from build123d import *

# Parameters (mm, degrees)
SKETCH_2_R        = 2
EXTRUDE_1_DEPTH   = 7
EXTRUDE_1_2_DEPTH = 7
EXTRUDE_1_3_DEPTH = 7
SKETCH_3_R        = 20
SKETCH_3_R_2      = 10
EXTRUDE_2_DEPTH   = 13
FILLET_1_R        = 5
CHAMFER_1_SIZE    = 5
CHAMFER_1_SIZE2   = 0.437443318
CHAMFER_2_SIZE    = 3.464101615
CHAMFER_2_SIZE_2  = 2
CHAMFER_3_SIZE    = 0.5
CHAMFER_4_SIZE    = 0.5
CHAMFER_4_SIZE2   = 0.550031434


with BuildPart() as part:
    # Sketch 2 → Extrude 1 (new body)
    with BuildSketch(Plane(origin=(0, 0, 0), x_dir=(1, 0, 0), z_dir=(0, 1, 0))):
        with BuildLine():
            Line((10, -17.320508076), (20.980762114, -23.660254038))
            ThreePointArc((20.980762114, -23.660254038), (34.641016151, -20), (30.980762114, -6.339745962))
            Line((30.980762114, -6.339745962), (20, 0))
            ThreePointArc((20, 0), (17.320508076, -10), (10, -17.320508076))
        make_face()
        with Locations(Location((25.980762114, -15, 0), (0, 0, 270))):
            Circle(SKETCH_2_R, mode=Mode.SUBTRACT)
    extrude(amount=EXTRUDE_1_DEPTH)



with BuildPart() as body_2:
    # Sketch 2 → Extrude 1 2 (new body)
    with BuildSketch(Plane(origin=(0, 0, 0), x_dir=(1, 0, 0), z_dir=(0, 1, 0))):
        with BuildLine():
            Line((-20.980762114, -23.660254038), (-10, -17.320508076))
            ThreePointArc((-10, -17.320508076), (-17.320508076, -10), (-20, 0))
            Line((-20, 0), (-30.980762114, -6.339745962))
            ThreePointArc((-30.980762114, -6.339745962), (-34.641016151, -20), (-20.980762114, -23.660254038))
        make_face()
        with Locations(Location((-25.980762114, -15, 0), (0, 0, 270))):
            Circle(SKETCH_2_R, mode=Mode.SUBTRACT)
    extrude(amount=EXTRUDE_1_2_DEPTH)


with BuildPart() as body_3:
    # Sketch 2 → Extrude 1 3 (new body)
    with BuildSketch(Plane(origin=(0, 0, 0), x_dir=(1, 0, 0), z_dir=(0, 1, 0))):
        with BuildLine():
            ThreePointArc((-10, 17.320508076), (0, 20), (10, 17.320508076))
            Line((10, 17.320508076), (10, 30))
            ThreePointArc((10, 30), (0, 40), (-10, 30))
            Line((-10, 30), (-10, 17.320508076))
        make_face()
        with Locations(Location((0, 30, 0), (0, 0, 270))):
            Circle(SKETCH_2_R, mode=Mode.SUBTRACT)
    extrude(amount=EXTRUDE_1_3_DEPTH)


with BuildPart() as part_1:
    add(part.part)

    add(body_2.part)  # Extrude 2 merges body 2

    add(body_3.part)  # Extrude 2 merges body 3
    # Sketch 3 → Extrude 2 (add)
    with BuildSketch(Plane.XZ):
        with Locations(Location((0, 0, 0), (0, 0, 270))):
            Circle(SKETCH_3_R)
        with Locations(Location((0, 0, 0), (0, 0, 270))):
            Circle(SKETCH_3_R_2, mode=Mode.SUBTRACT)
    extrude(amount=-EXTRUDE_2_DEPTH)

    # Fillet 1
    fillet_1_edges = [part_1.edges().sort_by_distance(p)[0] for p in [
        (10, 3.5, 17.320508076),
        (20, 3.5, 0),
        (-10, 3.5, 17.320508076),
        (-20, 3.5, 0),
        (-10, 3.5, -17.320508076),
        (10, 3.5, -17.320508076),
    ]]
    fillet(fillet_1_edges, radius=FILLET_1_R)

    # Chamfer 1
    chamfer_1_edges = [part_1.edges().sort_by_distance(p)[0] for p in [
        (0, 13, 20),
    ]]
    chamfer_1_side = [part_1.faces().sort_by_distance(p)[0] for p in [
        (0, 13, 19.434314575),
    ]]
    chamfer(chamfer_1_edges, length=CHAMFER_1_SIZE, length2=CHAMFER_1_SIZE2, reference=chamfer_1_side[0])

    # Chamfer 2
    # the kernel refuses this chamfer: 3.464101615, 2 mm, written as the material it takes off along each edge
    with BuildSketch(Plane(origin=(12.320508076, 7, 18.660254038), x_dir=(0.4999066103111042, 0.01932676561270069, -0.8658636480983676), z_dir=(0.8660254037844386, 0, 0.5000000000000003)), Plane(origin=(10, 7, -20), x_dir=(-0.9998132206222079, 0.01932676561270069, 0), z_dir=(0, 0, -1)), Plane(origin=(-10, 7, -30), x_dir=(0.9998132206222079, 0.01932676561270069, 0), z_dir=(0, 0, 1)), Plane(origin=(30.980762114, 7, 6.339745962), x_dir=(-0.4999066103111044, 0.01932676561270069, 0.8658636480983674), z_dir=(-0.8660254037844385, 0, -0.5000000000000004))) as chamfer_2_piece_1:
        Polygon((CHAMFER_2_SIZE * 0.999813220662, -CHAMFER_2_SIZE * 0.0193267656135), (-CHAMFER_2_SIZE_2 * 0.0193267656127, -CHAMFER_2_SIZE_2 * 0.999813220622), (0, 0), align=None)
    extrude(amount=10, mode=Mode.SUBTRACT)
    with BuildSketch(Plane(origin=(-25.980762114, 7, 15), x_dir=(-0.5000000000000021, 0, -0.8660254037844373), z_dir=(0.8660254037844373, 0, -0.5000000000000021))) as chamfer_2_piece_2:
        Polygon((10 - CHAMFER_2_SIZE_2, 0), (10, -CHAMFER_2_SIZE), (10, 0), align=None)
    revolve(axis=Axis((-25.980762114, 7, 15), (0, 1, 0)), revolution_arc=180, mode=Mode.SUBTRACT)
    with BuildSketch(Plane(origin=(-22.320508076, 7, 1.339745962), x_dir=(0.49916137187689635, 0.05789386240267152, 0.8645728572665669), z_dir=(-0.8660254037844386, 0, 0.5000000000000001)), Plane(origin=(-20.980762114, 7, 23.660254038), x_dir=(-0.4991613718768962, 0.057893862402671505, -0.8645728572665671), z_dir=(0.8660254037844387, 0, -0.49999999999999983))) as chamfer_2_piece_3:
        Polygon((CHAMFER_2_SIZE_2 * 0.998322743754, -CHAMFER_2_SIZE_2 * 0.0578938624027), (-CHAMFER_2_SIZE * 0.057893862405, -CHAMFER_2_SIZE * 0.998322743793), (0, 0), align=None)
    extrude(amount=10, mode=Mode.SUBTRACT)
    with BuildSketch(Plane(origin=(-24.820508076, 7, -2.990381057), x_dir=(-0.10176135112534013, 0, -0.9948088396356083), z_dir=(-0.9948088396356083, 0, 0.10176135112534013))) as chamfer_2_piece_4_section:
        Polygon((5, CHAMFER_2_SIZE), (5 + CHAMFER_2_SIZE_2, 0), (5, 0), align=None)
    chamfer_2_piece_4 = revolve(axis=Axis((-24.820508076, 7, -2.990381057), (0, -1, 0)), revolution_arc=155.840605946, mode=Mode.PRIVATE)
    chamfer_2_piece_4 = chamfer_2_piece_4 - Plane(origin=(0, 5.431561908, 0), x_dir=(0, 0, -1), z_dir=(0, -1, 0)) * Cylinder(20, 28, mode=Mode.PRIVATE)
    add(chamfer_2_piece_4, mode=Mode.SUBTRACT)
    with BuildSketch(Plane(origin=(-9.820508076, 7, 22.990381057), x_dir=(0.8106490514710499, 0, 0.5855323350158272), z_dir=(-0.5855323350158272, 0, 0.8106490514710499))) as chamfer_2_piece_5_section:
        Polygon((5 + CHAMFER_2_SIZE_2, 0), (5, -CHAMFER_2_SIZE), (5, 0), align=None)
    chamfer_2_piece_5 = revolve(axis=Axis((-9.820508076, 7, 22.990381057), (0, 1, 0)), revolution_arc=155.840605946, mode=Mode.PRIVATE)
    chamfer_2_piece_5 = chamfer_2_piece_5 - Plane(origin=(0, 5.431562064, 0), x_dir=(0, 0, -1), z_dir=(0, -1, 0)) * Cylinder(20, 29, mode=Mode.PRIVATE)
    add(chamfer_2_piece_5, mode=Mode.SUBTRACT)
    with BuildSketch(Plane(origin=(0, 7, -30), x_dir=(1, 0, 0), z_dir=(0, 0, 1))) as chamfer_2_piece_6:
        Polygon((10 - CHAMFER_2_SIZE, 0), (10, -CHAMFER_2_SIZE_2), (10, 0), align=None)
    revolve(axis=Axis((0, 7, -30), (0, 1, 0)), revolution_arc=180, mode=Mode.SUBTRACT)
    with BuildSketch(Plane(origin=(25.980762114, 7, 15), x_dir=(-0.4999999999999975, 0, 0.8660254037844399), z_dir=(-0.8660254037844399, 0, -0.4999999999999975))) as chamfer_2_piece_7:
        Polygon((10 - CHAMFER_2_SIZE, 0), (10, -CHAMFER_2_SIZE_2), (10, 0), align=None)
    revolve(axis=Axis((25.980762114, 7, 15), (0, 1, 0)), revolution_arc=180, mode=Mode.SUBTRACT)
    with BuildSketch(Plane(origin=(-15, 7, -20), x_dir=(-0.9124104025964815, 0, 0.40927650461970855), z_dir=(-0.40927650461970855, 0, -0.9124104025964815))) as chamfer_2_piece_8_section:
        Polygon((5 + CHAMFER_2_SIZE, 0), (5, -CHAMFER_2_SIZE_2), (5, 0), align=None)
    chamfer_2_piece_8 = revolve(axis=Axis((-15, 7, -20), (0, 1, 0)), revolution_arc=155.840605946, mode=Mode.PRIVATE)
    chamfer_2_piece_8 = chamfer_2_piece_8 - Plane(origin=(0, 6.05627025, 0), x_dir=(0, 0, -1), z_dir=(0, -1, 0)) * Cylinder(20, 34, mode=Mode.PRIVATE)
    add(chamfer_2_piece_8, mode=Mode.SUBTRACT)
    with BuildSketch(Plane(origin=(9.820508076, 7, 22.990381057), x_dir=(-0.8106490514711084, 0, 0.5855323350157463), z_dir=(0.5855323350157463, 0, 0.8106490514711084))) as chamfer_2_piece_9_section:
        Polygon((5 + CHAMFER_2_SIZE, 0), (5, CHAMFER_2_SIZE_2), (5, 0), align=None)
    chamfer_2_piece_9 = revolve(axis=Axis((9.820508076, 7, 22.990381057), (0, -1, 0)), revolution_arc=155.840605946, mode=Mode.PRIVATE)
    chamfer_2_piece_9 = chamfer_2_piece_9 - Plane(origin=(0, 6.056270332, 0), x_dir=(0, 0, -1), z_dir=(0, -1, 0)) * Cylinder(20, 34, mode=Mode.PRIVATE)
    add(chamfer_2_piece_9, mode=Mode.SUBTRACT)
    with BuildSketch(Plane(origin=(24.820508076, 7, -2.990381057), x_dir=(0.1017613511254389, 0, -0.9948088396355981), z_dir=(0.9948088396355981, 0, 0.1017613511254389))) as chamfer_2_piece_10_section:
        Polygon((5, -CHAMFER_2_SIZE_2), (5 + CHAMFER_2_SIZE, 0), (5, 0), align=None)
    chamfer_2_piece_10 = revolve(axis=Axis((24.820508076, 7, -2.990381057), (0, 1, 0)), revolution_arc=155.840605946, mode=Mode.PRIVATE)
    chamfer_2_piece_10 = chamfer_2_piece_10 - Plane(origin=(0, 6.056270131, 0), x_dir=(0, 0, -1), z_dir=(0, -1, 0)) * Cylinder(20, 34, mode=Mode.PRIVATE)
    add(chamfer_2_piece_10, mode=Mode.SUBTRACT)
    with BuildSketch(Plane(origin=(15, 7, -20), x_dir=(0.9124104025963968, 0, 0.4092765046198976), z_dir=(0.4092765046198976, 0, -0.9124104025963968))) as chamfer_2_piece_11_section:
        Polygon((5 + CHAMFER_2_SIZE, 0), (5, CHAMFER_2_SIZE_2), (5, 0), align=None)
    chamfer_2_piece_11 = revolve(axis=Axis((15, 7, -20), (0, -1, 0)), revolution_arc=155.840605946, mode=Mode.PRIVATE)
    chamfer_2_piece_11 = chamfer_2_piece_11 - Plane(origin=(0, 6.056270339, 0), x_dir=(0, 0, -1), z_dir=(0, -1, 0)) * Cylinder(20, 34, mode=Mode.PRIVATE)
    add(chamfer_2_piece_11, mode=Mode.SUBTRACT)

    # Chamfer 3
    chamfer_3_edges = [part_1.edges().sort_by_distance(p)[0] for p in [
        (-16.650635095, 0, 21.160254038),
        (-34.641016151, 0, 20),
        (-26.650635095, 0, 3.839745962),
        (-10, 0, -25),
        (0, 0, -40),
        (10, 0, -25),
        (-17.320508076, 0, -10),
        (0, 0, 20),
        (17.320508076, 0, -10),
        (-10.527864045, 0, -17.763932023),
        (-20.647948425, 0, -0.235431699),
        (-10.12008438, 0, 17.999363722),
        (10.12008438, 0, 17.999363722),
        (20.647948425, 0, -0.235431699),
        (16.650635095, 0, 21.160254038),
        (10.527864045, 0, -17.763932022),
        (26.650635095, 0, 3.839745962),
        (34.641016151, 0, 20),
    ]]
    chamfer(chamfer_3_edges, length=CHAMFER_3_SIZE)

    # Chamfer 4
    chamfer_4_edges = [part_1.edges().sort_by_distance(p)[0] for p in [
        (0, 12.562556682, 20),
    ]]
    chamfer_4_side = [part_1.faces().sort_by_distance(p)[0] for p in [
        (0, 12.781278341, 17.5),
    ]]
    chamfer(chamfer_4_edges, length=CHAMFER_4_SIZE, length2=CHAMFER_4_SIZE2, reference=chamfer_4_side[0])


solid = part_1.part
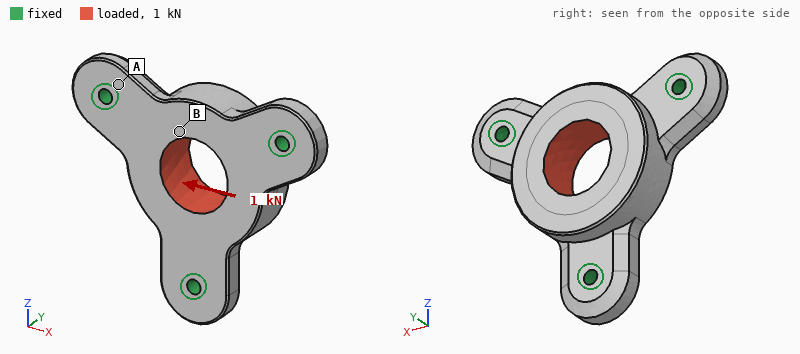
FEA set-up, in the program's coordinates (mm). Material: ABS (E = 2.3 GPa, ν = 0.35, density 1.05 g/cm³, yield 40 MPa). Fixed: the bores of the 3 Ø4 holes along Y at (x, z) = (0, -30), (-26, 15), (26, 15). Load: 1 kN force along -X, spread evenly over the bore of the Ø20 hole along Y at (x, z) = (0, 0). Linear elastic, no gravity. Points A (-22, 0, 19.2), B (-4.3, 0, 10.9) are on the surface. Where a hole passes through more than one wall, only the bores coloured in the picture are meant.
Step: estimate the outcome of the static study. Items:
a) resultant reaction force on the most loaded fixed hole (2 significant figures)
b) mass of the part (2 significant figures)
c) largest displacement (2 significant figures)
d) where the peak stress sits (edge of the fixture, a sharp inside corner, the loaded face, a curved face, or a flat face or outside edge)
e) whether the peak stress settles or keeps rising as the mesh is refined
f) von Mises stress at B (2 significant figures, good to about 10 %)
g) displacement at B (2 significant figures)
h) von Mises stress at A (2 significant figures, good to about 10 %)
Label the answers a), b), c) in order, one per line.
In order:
a) 430 N
b) 20 g
c) 0.10 mm
d) edge of the fixture
e) keeps rising
f) 4.2 MPa
g) 0.034 mm
h) 1.8 MPa
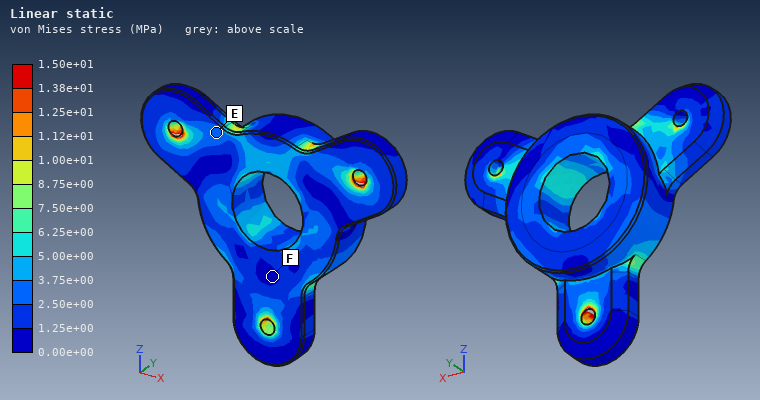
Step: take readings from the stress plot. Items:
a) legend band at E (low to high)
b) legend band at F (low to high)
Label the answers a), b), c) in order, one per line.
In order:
a) 2.50e+00 to 3.75e+00 MPa
b) 0.00e+00 to 1.25e+00 MPa
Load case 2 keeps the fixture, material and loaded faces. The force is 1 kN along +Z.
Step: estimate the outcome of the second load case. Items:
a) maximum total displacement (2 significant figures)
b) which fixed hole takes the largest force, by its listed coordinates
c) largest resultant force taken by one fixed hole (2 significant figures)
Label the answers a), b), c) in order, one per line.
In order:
a) 0.11 mm
b) (0, -30)
c) 490 N
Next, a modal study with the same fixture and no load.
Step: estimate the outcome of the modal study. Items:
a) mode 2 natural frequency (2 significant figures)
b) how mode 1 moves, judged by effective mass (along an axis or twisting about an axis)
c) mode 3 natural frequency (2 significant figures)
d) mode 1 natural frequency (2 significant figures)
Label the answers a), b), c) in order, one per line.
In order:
a) 4500 Hz
b) along Y
c) 4500 Hz
d) 3500 Hz
